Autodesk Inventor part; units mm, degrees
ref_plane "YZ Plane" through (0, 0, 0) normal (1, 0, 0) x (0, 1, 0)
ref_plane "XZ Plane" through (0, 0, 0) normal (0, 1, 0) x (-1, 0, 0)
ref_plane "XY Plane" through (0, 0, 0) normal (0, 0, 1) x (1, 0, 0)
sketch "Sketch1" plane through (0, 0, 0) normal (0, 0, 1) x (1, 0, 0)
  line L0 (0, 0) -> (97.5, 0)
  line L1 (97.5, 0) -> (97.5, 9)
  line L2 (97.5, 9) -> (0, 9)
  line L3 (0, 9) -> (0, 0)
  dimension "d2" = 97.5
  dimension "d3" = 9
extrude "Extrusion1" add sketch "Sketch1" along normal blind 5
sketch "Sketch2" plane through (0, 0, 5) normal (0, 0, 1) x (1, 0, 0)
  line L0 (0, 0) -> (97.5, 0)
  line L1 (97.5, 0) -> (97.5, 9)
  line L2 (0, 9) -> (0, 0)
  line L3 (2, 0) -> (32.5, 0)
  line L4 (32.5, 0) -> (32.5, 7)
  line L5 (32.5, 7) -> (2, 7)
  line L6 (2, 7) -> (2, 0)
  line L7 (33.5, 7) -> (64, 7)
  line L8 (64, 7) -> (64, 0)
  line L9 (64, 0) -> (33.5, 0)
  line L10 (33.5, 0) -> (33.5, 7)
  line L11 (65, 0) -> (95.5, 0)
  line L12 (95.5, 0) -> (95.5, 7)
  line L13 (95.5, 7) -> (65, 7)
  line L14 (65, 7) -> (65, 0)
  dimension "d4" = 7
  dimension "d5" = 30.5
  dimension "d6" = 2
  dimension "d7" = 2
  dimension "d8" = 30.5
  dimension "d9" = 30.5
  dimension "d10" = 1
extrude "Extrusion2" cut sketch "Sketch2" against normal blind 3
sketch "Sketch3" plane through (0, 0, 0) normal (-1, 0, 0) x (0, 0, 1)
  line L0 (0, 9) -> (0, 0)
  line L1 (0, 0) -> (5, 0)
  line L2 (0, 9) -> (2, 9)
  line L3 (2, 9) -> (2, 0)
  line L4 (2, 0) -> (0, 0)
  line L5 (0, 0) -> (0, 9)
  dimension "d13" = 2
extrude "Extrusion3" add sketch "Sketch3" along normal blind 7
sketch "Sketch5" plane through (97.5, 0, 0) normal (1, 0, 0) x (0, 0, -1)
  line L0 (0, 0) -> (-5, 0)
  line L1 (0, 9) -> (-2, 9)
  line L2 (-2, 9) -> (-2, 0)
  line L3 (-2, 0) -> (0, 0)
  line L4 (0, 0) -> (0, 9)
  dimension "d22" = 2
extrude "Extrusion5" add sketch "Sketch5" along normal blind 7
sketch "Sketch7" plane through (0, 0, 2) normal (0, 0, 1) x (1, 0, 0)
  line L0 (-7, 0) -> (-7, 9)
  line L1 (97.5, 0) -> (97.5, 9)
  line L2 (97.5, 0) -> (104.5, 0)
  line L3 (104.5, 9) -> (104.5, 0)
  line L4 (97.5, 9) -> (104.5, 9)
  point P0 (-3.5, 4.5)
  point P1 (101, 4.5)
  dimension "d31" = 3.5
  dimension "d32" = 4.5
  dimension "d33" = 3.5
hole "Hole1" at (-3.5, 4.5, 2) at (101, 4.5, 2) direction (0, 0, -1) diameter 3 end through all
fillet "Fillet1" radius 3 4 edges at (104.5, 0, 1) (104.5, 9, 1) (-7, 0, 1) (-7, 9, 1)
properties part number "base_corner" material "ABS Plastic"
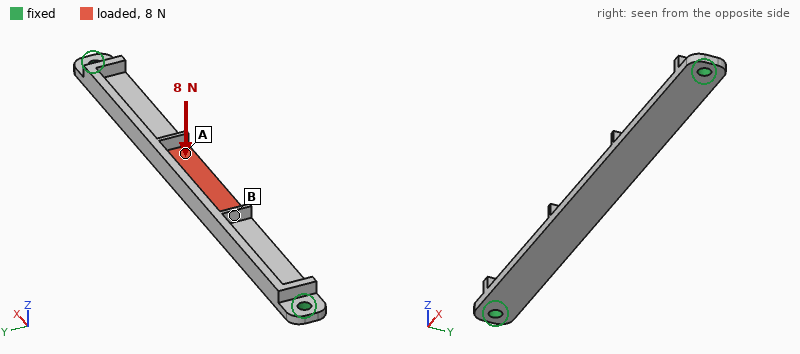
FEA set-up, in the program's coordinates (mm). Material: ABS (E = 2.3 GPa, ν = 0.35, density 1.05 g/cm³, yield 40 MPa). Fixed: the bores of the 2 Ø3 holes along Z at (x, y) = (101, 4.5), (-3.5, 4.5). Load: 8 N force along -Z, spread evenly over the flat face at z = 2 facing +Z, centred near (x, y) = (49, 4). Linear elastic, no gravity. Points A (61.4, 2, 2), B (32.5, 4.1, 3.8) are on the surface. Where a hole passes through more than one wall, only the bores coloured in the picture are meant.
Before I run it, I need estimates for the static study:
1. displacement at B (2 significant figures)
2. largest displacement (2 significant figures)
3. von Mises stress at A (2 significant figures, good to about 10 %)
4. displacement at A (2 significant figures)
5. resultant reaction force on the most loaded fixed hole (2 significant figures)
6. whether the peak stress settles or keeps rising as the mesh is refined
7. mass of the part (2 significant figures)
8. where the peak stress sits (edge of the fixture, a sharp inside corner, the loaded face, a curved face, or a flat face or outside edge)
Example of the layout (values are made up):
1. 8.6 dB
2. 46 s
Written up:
1. 0.82 mm
2. 1.1 mm
3. 3.2 MPa
4. 0.92 mm
5. 11 N
6. keeps rising
7. 2.8 g
8. edge of the fixture
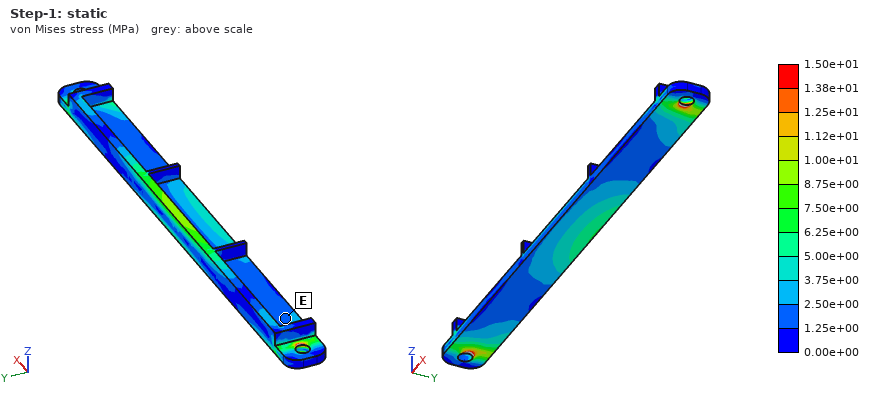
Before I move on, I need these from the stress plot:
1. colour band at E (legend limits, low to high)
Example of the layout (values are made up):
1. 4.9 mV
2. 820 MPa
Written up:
1. 1.25e+00 to 2.50e+00 MPa
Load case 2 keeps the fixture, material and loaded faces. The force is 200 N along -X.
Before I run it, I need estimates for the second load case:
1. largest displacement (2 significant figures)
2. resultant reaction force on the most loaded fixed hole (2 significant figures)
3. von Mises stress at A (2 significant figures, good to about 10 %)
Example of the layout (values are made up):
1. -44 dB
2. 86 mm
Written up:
1. 0.17 mm
2. 100 N
3. 8.0 MPa
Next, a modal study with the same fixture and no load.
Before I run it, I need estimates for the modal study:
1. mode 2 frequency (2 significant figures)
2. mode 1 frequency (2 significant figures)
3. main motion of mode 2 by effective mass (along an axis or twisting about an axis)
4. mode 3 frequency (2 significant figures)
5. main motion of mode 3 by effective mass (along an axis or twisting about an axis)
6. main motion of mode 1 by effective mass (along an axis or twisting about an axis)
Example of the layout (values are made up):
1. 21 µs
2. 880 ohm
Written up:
1. 980 Hz
2. 420 Hz
3. along Y
4. 1200 Hz
5. twisting about Y
6. along Z
